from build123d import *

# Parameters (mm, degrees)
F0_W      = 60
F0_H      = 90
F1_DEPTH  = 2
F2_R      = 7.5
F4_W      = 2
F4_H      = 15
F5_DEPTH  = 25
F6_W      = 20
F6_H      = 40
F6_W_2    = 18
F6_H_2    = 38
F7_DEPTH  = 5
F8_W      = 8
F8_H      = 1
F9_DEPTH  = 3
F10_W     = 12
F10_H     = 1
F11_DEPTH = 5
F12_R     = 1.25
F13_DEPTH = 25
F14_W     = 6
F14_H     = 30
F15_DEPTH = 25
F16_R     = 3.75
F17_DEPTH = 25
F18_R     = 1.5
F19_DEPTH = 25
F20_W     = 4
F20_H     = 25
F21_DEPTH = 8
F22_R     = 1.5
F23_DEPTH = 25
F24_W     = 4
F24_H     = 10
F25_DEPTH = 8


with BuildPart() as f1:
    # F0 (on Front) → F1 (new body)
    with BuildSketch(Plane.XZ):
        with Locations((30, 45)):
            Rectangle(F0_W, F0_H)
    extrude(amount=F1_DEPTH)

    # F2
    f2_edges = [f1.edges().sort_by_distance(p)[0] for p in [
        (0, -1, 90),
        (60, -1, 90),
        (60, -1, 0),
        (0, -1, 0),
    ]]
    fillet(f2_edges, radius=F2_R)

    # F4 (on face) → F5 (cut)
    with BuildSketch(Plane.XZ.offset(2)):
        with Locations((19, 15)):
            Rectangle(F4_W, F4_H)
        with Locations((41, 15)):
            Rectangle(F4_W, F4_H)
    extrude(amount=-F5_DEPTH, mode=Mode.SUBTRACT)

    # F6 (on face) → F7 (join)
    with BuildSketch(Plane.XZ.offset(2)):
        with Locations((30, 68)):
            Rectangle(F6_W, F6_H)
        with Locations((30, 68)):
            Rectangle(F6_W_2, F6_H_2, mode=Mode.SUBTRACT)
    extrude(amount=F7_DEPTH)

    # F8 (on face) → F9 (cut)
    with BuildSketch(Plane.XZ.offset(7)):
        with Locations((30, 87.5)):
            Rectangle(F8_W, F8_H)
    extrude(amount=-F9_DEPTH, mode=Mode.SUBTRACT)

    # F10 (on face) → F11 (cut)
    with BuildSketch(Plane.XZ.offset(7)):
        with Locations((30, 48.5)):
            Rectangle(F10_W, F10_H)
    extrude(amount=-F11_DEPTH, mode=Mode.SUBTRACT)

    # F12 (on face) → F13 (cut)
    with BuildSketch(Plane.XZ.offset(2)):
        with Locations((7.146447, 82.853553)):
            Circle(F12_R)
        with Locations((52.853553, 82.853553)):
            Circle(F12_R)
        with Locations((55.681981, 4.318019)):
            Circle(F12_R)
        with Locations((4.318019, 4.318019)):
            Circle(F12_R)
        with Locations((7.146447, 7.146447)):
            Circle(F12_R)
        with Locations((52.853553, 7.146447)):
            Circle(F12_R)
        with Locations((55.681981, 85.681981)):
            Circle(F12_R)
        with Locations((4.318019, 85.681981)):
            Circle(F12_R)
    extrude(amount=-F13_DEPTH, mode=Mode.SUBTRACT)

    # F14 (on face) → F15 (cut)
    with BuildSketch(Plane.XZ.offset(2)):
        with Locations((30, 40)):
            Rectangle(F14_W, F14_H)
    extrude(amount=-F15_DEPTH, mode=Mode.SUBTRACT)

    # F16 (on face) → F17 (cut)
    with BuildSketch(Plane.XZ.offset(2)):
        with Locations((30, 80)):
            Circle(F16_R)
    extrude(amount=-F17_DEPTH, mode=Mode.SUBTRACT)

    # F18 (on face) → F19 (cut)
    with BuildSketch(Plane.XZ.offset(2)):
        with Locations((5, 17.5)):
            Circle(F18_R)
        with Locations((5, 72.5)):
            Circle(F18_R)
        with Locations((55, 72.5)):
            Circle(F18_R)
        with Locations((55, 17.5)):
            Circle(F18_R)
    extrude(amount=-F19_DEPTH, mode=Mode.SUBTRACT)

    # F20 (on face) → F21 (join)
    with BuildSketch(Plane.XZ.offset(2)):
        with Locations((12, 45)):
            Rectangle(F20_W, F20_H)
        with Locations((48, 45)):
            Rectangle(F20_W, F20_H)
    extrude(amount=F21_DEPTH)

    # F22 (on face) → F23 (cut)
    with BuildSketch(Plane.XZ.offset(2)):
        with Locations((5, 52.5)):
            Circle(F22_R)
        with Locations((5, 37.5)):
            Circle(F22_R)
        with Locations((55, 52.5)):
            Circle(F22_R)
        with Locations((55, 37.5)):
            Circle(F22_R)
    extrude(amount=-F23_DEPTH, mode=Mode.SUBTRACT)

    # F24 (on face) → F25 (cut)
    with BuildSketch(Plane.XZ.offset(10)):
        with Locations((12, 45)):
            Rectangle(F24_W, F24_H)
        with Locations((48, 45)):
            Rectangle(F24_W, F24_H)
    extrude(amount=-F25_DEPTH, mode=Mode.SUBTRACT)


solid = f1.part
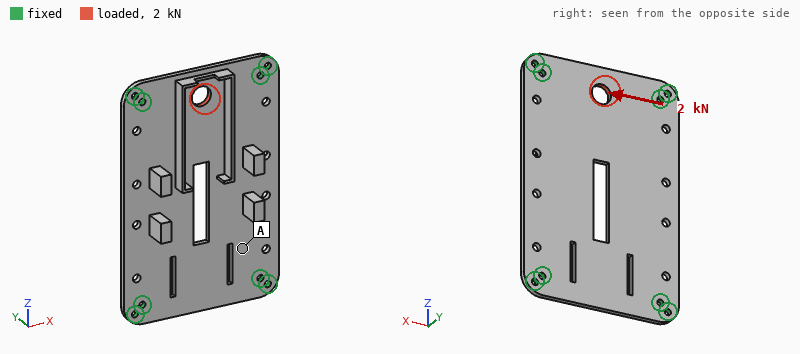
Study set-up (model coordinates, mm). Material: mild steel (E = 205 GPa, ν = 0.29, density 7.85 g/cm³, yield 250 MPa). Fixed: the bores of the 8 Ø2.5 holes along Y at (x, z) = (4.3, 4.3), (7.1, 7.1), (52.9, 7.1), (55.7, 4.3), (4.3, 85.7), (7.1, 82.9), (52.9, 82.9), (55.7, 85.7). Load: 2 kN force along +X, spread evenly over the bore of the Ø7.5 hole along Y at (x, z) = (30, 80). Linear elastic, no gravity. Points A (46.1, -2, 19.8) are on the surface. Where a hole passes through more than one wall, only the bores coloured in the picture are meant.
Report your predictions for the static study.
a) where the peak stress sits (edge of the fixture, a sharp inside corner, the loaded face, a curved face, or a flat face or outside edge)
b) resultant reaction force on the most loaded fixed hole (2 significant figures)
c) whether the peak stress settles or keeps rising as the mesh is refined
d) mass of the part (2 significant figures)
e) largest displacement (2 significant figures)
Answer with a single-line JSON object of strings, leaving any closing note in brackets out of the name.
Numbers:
{"where the peak stress sits": "edge of the fixture", "resultant reaction force on the most loaded fixed hole": "710 N", "whether the peak stress settles or keeps rising as the mesh is refined": "keeps rising", "mass of the part": "89 g", "largest displacement": "4.0 µm"}
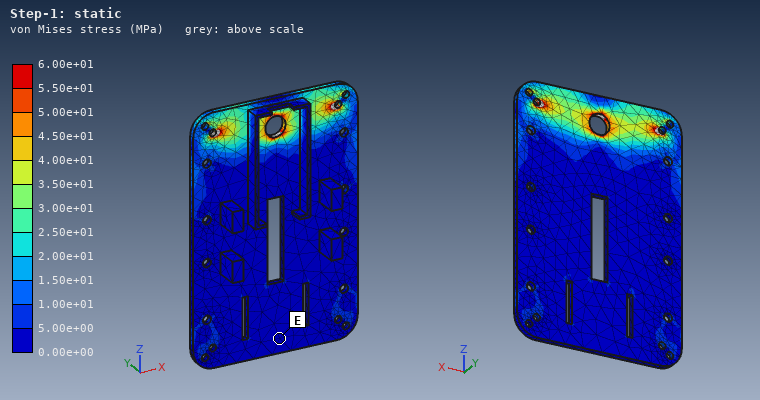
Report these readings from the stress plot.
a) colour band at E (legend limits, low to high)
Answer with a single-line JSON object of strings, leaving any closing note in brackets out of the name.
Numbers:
{"colour band at E": "0.00e+00 to 5.00e+00 MPa"}
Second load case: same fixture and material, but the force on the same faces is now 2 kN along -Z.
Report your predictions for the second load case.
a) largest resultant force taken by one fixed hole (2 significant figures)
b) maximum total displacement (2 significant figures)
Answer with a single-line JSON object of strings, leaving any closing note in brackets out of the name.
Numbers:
{"largest resultant force taken by one fixed hole": "610 N", "maximum total displacement": "8.1 µm"}
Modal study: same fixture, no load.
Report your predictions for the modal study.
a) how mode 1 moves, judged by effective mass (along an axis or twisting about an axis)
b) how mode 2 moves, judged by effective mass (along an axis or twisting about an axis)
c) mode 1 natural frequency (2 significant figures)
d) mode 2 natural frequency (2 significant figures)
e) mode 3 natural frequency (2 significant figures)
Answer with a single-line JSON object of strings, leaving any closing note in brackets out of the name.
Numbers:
{"how mode 1 moves, judged by effective mass": "along Y", "how mode 2 moves, judged by effective mass": "twisting about Z", "mode 1 natural frequency": "1500 Hz", "mode 2 natural frequency": "2100 Hz", "mode 3 natural frequency": "3300 Hz"}
